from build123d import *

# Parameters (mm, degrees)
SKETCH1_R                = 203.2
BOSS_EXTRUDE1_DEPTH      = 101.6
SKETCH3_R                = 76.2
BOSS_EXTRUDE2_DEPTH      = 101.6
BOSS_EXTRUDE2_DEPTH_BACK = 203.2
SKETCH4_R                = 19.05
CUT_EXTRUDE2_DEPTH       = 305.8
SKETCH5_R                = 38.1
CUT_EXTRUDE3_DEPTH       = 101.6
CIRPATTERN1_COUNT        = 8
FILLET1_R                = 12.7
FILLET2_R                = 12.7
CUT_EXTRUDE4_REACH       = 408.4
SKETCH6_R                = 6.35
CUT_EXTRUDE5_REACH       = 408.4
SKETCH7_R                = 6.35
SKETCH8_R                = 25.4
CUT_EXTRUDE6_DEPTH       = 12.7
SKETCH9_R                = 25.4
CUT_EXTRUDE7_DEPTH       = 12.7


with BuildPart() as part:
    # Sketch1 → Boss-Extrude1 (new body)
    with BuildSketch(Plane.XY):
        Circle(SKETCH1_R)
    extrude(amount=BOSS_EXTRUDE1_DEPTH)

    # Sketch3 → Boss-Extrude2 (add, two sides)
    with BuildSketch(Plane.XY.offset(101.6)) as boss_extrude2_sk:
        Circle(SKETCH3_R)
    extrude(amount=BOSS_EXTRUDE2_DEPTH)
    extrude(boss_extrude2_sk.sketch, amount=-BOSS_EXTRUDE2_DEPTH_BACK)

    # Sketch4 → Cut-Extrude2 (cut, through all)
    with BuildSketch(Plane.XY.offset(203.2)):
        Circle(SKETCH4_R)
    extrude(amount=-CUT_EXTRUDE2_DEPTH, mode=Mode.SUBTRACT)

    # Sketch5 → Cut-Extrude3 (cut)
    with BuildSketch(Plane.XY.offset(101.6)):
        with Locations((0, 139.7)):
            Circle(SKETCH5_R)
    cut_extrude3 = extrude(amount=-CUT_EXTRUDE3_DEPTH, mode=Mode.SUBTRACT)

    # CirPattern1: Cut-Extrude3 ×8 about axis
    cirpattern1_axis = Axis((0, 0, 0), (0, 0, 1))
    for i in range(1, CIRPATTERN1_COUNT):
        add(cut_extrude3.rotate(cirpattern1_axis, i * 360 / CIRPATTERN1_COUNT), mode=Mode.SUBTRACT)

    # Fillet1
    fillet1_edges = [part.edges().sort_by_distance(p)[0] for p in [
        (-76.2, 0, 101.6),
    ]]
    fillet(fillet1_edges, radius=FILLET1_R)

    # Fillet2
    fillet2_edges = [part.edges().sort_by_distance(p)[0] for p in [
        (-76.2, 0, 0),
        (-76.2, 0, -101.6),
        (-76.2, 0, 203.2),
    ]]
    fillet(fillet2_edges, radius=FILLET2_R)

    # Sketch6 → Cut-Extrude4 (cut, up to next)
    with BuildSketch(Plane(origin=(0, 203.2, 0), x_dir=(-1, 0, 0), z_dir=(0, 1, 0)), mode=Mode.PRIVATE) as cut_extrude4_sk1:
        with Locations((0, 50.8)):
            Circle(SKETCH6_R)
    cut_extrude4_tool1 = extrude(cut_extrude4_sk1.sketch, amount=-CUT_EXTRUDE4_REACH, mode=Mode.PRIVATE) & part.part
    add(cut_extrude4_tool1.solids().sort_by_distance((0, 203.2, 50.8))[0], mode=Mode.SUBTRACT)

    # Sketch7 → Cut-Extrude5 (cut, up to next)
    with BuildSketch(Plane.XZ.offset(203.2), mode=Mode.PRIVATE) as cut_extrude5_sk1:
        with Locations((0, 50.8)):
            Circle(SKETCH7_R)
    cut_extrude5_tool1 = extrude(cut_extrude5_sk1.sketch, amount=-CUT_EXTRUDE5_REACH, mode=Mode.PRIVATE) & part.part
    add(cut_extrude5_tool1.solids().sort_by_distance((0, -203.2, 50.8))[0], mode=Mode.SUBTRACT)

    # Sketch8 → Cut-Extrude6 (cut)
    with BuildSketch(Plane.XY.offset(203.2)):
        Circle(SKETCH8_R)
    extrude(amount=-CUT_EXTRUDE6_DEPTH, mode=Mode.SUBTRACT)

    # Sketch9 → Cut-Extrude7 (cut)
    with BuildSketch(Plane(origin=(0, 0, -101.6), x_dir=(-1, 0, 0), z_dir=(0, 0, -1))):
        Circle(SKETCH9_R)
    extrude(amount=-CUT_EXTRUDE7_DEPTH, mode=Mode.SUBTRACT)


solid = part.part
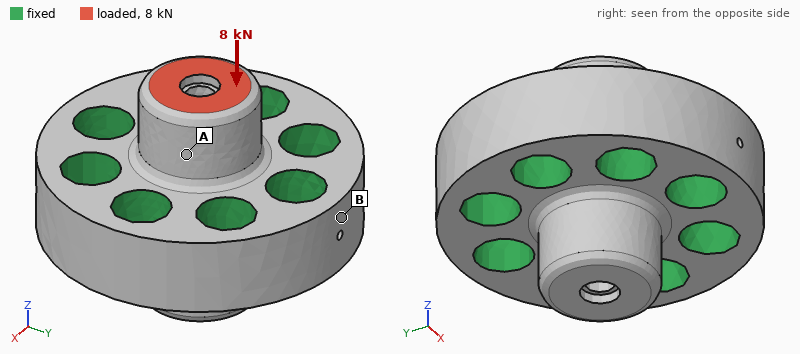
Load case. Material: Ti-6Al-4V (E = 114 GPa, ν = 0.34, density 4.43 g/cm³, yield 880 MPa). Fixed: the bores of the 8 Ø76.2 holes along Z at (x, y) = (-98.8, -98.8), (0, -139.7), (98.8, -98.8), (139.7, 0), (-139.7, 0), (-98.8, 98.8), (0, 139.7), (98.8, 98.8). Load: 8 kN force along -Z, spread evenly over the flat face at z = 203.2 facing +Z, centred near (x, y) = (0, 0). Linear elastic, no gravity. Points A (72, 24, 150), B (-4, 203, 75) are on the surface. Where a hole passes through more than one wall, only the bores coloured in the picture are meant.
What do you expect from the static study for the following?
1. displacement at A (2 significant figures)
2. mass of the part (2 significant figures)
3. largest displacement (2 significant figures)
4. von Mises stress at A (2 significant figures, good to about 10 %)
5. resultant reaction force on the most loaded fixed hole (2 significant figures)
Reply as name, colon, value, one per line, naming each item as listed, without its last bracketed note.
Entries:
displacement at A: 0.41 µm
mass of the part: 57 kg
largest displacement: 0.70 µm
von Mises stress at A: 0.38 MPa
resultant reaction force on the most loaded fixed hole: 1.2 kN
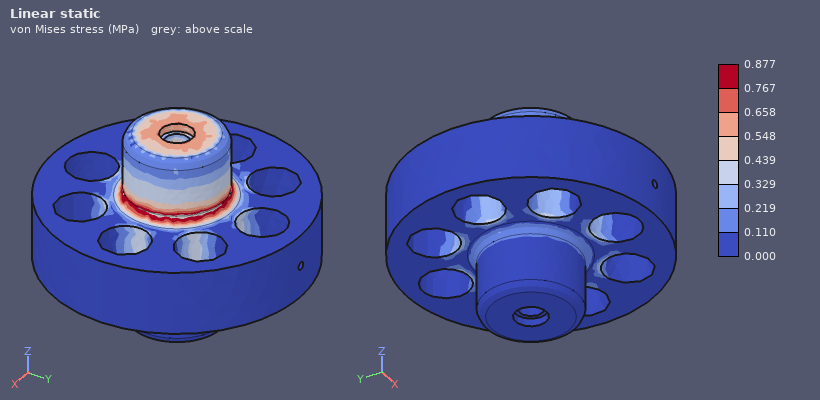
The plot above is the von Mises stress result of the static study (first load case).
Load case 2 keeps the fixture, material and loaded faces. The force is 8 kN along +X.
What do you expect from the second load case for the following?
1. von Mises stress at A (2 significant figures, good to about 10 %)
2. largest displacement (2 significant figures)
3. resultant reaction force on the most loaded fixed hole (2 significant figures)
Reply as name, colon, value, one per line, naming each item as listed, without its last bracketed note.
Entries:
von Mises stress at A: 1.3 MPa
largest displacement: 3.6 µm
resultant reaction force on the most loaded fixed hole: 3.3 kN
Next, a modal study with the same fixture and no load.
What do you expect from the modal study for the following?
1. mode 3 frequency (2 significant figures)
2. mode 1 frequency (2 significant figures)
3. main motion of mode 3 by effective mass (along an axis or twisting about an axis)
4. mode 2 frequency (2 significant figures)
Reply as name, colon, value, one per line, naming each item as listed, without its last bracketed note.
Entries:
mode 3 frequency: 4900 Hz
mode 1 frequency: 4500 Hz
main motion of mode 3 by effective mass: along Y
mode 2 frequency: 4500 Hz
